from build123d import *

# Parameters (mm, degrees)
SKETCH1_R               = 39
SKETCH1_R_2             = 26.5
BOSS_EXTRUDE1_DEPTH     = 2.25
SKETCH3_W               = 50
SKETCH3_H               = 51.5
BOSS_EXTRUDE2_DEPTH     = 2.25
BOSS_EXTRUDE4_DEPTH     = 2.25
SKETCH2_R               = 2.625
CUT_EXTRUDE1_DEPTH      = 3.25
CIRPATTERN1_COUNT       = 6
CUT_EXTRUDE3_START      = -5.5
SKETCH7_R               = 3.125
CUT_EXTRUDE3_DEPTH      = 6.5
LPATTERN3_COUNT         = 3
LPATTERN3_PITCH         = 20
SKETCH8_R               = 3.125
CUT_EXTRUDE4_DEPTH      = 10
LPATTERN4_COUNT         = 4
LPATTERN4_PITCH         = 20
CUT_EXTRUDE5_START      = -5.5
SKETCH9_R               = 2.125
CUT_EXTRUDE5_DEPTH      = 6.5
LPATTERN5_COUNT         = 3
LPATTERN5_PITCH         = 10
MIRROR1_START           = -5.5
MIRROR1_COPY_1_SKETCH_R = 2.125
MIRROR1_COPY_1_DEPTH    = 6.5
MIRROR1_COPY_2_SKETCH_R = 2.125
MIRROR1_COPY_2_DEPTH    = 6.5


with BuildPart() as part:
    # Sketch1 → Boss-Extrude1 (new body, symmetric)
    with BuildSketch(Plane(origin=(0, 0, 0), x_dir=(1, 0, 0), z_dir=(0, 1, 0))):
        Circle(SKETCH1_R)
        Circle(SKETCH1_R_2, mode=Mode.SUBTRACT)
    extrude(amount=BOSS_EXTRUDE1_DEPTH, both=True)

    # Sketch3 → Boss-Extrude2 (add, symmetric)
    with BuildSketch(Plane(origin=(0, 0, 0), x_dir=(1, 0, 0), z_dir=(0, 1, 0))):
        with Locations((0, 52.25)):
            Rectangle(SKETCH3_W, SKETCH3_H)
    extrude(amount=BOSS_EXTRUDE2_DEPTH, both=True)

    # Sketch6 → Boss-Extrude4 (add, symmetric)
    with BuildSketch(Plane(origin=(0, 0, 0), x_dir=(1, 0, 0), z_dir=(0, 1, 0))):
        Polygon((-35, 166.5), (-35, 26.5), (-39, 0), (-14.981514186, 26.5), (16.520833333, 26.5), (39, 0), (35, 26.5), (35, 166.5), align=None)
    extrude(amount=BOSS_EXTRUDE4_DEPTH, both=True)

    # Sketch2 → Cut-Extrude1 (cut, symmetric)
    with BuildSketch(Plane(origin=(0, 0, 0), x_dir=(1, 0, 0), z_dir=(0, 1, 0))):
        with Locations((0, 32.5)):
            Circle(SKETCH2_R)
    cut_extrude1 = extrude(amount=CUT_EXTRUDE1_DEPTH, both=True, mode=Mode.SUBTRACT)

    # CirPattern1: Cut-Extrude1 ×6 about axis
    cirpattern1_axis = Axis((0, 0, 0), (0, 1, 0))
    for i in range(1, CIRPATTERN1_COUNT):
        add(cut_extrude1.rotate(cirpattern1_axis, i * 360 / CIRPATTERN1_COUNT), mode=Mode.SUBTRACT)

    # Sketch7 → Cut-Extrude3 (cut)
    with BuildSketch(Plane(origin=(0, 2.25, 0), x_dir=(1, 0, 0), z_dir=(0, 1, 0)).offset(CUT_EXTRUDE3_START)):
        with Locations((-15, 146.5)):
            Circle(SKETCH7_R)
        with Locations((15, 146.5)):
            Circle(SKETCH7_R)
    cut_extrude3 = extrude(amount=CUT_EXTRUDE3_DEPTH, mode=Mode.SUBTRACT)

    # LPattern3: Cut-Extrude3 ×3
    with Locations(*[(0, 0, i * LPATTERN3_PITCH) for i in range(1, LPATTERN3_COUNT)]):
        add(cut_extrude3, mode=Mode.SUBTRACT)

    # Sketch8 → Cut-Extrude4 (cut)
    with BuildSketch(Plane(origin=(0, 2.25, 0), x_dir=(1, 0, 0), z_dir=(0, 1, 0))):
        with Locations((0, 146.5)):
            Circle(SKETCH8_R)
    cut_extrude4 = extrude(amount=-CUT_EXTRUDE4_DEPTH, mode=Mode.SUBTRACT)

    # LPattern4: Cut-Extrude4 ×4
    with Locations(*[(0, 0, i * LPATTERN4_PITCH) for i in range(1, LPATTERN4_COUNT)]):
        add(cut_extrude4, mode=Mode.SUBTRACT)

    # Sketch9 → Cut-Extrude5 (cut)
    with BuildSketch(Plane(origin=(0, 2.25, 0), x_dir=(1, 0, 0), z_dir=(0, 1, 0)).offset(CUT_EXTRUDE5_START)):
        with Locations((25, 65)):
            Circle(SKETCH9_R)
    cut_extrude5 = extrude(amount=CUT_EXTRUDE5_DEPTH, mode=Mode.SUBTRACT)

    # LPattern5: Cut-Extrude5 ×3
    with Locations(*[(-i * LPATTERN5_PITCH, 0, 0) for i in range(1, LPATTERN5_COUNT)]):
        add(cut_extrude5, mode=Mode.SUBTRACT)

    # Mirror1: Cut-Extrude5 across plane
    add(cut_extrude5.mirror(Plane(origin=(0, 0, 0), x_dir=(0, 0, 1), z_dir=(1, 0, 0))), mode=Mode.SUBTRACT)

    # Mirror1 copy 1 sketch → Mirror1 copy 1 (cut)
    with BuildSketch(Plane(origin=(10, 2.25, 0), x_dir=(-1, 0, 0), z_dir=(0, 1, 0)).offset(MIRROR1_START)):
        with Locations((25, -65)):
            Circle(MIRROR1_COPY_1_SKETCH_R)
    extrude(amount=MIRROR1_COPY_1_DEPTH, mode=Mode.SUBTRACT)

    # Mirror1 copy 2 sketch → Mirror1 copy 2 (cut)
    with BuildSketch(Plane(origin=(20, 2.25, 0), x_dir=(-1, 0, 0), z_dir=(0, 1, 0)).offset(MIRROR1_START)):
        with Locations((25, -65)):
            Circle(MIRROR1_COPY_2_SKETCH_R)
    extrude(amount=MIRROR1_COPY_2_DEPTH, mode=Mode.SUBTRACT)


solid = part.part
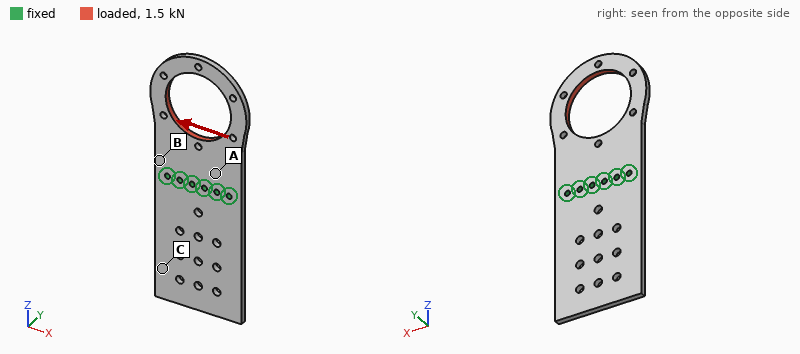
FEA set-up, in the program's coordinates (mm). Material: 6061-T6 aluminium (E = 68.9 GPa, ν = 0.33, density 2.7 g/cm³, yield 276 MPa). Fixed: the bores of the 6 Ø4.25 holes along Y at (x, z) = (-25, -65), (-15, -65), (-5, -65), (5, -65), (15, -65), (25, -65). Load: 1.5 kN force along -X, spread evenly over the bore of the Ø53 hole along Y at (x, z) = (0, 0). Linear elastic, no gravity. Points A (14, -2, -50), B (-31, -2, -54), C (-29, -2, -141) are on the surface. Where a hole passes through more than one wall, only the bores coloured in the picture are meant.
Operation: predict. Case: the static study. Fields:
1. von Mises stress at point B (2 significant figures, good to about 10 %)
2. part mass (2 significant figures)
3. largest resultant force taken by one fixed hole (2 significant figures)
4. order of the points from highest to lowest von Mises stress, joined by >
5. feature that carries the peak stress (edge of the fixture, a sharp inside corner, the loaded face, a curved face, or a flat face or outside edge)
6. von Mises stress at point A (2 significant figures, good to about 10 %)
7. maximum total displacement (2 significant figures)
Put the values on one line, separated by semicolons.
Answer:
21 MPa; 140 g; 1.6 kN; B > A > C; the loaded face; 12 MPa; 0.15 mm
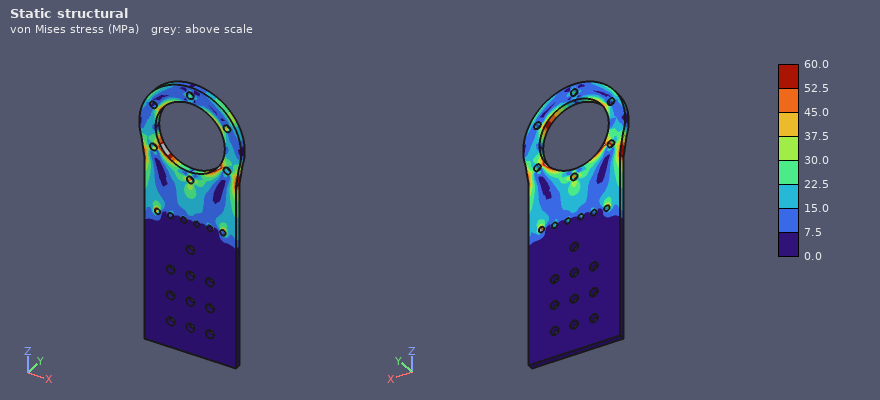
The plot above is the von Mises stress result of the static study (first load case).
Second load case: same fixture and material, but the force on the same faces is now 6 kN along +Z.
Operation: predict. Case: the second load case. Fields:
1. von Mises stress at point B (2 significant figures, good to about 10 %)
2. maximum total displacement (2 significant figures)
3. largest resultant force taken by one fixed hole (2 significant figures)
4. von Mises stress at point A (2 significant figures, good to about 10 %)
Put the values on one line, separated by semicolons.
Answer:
29 MPa; 0.10 mm; 1.6 kN; 15 MPa
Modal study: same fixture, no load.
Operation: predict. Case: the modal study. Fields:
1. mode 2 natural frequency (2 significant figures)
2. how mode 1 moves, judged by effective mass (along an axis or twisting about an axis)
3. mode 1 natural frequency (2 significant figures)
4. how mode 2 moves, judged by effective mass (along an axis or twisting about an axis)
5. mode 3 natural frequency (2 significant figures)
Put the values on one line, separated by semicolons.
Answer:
440 Hz; along Y; 370 Hz; along Y; 1100 Hz
